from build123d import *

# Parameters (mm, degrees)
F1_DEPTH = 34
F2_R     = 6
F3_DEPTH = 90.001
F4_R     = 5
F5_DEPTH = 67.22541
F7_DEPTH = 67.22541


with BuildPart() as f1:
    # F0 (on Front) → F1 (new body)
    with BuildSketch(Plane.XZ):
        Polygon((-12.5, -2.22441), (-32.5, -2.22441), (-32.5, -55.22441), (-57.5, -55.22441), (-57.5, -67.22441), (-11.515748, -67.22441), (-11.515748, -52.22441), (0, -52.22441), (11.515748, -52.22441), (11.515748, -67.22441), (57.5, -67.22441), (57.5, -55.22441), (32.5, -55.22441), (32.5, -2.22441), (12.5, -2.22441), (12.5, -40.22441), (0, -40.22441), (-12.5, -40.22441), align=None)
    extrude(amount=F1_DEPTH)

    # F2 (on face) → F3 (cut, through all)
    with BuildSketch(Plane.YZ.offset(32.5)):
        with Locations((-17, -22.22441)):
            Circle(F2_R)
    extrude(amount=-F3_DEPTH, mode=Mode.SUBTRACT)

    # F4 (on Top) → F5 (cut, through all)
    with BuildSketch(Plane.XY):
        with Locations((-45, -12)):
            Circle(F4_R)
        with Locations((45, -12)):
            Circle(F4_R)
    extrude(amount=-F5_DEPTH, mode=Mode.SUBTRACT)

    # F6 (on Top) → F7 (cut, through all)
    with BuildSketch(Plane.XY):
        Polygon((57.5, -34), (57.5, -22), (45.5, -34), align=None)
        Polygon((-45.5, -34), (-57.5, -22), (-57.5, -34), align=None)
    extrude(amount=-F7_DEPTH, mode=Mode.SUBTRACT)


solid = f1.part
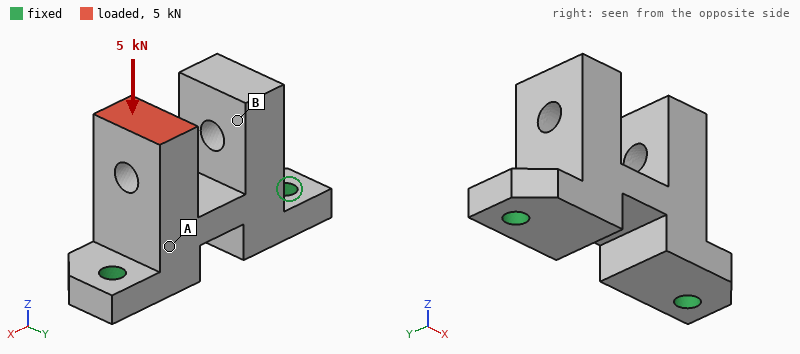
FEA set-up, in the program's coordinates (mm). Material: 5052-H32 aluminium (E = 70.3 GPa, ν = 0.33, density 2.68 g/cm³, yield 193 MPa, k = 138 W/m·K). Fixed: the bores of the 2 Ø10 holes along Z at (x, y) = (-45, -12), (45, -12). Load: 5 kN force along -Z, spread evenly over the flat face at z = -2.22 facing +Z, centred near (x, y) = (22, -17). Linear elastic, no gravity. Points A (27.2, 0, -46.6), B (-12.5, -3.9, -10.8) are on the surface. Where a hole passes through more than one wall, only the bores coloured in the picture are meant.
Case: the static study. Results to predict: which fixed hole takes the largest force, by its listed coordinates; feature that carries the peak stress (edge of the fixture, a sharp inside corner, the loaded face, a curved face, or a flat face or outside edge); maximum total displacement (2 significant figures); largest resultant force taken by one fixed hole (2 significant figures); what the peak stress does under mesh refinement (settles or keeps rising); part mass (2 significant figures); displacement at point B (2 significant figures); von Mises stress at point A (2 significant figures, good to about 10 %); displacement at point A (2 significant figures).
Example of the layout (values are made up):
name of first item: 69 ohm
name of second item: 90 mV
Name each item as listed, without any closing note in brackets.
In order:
which fixed hole takes the largest force, by its listed coordinates: (45, -12)
feature that carries the peak stress: edge of the fixture
maximum total displacement: 36 µm
largest resultant force taken by one fixed hole: 4.5 kN
what the peak stress does under mesh refinement: keeps rising
part mass: 300 g
displacement at point B: 17 µm
von Mises stress at point A: 13 MPa
displacement at point A: 11 µm
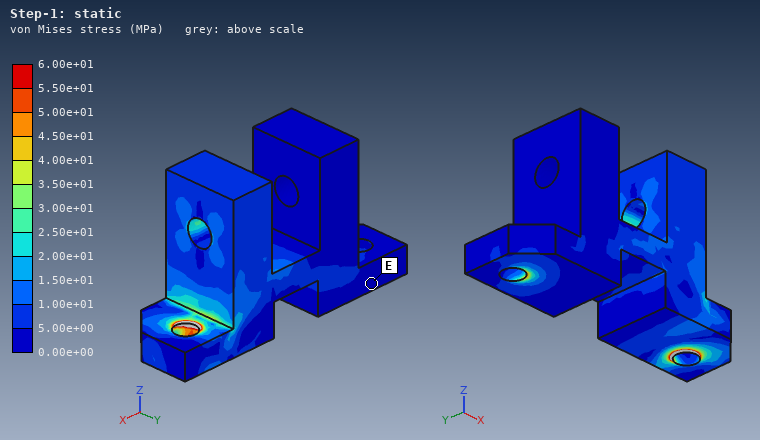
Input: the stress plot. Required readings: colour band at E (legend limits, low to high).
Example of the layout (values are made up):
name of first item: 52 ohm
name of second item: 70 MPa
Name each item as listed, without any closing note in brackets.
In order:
colour band at E: 0.00e+00 to 5.00e+00 MPa
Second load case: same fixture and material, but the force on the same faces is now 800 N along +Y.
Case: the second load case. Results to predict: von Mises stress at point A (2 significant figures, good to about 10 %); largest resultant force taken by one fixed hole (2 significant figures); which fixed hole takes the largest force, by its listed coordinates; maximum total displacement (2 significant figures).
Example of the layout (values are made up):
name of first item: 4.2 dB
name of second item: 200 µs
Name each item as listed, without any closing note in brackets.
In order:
von Mises stress at point A: 10 MPa
largest resultant force taken by one fixed hole: 530 N
which fixed hole takes the largest force, by its listed coordinates: (45, -12)
maximum total displacement: 77 µm
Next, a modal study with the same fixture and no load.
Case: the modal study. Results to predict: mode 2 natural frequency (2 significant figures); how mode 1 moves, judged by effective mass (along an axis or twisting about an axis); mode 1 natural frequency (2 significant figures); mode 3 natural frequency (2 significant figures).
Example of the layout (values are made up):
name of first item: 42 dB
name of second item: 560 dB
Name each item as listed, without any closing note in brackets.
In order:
mode 2 natural frequency: 4000 Hz
how mode 1 moves, judged by effective mass: along Y
mode 1 natural frequency: 2200 Hz
mode 3 natural frequency: 4900 Hz
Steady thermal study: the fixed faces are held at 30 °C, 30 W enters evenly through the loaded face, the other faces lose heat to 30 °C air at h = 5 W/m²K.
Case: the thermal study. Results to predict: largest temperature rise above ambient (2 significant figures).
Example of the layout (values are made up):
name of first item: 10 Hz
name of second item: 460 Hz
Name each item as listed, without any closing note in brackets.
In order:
largest temperature rise above ambient: 25 K
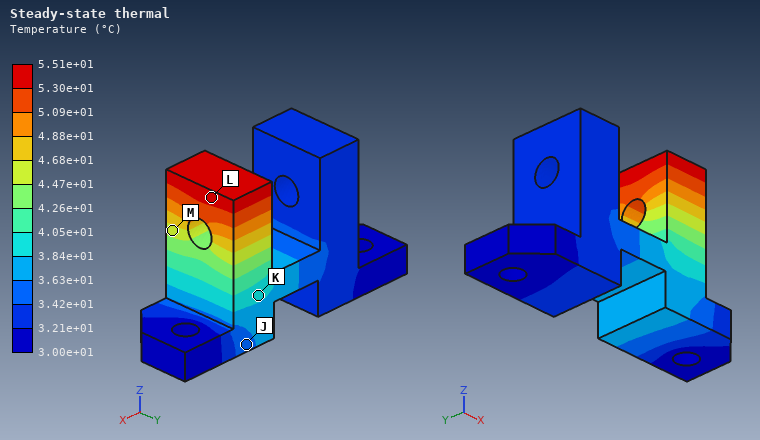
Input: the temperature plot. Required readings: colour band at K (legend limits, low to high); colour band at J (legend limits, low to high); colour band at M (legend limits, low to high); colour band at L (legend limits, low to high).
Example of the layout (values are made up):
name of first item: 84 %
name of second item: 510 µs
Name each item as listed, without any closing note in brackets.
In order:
colour band at K: 3.84e+01 to 4.05e+01 °C
colour band at J: 3.42e+01 to 3.63e+01 °C
colour band at M: 4.47e+01 to 4.68e+01 °C
colour band at L: 5.30e+01 to 5.51e+01 °C
